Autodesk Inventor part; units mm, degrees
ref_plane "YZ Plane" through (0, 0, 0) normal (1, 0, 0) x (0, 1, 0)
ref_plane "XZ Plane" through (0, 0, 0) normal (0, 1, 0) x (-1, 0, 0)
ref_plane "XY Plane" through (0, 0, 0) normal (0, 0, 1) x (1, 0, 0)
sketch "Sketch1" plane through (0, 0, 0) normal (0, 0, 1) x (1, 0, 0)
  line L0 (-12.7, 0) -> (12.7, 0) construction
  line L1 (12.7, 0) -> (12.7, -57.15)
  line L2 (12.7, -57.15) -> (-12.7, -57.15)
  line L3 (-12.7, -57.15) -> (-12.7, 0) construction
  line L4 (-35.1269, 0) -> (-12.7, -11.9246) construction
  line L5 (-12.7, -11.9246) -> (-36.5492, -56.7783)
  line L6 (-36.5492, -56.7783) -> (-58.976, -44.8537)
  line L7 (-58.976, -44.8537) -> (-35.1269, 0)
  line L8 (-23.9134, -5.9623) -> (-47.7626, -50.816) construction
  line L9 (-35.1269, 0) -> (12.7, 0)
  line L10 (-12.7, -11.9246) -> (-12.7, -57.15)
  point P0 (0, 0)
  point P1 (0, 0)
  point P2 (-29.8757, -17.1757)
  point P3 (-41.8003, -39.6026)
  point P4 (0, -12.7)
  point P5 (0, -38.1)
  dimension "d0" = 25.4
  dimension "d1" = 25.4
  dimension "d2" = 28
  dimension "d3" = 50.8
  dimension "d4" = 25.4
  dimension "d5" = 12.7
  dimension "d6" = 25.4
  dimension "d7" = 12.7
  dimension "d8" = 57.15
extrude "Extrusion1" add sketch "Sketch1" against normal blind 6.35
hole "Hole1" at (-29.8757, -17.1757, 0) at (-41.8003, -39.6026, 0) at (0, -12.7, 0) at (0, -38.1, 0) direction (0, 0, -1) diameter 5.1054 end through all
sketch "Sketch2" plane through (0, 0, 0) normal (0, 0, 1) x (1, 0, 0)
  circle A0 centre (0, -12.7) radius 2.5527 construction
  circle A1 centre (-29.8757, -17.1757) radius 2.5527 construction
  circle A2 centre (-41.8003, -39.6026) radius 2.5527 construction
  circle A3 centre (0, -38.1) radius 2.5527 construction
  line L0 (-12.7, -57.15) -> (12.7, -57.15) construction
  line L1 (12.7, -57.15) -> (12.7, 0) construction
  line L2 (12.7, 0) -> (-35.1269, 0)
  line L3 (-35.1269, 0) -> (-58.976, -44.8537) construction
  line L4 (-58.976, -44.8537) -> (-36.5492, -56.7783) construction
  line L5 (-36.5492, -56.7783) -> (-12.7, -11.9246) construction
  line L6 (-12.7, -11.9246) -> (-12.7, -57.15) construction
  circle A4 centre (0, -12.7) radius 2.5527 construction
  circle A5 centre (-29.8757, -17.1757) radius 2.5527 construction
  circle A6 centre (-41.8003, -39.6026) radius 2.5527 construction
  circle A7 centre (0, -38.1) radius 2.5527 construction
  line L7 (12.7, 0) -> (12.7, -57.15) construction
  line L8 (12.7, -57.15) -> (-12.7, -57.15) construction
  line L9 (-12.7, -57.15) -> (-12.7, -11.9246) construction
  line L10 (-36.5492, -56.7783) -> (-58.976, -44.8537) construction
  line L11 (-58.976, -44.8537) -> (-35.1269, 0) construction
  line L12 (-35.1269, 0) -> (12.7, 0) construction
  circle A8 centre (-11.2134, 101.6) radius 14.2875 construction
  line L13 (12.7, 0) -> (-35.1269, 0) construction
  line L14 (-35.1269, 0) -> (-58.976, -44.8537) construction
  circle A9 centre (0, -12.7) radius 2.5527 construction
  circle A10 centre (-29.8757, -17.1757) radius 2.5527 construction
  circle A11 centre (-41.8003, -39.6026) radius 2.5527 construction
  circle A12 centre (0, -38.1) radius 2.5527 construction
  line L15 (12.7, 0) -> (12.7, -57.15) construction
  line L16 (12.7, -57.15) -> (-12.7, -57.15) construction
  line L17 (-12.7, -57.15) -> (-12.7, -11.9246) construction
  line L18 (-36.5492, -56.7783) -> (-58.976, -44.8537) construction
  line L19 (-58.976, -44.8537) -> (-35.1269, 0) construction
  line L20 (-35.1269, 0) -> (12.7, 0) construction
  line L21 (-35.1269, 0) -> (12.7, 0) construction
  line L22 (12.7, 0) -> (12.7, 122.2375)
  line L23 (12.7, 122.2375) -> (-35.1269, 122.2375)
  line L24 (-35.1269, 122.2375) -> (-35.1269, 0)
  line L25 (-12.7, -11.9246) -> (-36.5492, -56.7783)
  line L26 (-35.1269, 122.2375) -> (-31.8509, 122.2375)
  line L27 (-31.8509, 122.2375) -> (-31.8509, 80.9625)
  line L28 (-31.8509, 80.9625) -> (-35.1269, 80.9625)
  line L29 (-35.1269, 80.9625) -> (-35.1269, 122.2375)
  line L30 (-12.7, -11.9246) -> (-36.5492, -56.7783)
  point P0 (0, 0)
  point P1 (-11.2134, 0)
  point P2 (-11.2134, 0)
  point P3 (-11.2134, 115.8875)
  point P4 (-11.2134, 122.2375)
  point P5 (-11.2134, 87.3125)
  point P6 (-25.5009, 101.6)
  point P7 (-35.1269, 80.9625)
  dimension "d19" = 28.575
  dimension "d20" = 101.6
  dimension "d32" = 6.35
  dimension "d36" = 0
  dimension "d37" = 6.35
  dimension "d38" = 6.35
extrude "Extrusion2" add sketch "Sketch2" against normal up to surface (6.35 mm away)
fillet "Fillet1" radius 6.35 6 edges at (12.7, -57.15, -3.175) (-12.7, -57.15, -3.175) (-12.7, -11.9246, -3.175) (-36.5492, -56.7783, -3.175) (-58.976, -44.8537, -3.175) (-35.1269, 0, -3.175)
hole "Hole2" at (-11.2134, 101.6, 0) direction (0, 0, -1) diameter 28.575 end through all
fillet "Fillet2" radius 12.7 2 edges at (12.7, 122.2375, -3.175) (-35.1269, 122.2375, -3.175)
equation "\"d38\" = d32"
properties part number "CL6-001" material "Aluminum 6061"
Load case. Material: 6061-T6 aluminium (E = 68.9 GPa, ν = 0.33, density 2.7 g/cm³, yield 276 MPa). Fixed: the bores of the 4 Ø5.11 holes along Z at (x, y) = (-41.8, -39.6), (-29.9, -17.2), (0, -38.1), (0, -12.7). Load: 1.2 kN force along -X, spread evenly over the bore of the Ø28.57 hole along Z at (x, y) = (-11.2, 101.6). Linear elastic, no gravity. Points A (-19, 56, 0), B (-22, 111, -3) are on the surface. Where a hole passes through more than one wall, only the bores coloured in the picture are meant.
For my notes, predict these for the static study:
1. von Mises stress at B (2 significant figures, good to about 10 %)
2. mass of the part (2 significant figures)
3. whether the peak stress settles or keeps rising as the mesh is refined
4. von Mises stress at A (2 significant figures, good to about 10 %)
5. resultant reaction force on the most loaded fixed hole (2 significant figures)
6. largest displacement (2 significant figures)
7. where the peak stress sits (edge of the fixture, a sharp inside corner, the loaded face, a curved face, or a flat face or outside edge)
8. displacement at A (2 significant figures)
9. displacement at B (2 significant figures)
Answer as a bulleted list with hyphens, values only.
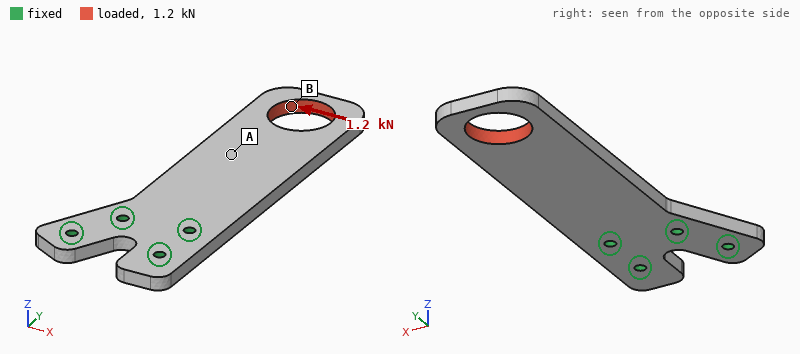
- 25 MPa
- 140 g
- keeps rising
- 12 MPa
- 3.3 kN
- 0.25 mm
- edge of the fixture
- 0.084 mm
- 0.22 mm
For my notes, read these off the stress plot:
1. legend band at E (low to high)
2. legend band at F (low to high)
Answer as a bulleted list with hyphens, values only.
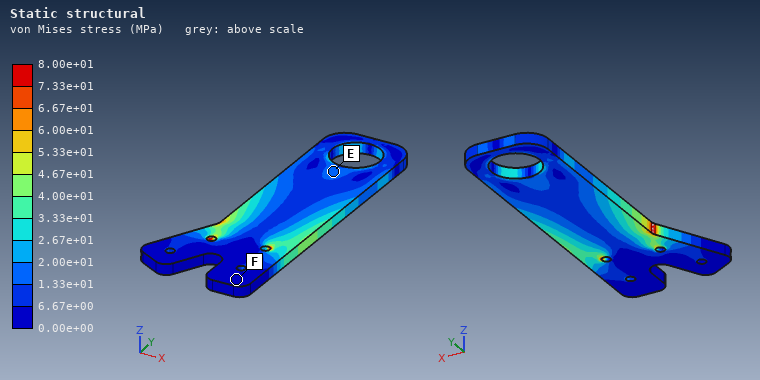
- 1.33e+01 to 2.00e+01 MPa
- 0.00e+00 to 6.67e+00 MPa
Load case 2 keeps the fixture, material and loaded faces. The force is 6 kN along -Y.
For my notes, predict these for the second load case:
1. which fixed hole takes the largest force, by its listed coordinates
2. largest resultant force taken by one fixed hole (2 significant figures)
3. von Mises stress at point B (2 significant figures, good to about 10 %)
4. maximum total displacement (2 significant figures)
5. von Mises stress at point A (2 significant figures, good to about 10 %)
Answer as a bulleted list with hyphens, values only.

- (0, -12.7)
- 3.0 kN
- 43 MPa
- 68 µm
- 18 MPa
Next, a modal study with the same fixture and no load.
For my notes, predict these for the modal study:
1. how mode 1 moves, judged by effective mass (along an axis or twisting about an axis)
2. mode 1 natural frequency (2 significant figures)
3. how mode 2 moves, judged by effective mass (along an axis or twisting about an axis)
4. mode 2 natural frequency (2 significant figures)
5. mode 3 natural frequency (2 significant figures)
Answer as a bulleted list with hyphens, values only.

- along Z
- 330 Hz
- twisting about Y
- 1600 Hz
- 1800 Hz
